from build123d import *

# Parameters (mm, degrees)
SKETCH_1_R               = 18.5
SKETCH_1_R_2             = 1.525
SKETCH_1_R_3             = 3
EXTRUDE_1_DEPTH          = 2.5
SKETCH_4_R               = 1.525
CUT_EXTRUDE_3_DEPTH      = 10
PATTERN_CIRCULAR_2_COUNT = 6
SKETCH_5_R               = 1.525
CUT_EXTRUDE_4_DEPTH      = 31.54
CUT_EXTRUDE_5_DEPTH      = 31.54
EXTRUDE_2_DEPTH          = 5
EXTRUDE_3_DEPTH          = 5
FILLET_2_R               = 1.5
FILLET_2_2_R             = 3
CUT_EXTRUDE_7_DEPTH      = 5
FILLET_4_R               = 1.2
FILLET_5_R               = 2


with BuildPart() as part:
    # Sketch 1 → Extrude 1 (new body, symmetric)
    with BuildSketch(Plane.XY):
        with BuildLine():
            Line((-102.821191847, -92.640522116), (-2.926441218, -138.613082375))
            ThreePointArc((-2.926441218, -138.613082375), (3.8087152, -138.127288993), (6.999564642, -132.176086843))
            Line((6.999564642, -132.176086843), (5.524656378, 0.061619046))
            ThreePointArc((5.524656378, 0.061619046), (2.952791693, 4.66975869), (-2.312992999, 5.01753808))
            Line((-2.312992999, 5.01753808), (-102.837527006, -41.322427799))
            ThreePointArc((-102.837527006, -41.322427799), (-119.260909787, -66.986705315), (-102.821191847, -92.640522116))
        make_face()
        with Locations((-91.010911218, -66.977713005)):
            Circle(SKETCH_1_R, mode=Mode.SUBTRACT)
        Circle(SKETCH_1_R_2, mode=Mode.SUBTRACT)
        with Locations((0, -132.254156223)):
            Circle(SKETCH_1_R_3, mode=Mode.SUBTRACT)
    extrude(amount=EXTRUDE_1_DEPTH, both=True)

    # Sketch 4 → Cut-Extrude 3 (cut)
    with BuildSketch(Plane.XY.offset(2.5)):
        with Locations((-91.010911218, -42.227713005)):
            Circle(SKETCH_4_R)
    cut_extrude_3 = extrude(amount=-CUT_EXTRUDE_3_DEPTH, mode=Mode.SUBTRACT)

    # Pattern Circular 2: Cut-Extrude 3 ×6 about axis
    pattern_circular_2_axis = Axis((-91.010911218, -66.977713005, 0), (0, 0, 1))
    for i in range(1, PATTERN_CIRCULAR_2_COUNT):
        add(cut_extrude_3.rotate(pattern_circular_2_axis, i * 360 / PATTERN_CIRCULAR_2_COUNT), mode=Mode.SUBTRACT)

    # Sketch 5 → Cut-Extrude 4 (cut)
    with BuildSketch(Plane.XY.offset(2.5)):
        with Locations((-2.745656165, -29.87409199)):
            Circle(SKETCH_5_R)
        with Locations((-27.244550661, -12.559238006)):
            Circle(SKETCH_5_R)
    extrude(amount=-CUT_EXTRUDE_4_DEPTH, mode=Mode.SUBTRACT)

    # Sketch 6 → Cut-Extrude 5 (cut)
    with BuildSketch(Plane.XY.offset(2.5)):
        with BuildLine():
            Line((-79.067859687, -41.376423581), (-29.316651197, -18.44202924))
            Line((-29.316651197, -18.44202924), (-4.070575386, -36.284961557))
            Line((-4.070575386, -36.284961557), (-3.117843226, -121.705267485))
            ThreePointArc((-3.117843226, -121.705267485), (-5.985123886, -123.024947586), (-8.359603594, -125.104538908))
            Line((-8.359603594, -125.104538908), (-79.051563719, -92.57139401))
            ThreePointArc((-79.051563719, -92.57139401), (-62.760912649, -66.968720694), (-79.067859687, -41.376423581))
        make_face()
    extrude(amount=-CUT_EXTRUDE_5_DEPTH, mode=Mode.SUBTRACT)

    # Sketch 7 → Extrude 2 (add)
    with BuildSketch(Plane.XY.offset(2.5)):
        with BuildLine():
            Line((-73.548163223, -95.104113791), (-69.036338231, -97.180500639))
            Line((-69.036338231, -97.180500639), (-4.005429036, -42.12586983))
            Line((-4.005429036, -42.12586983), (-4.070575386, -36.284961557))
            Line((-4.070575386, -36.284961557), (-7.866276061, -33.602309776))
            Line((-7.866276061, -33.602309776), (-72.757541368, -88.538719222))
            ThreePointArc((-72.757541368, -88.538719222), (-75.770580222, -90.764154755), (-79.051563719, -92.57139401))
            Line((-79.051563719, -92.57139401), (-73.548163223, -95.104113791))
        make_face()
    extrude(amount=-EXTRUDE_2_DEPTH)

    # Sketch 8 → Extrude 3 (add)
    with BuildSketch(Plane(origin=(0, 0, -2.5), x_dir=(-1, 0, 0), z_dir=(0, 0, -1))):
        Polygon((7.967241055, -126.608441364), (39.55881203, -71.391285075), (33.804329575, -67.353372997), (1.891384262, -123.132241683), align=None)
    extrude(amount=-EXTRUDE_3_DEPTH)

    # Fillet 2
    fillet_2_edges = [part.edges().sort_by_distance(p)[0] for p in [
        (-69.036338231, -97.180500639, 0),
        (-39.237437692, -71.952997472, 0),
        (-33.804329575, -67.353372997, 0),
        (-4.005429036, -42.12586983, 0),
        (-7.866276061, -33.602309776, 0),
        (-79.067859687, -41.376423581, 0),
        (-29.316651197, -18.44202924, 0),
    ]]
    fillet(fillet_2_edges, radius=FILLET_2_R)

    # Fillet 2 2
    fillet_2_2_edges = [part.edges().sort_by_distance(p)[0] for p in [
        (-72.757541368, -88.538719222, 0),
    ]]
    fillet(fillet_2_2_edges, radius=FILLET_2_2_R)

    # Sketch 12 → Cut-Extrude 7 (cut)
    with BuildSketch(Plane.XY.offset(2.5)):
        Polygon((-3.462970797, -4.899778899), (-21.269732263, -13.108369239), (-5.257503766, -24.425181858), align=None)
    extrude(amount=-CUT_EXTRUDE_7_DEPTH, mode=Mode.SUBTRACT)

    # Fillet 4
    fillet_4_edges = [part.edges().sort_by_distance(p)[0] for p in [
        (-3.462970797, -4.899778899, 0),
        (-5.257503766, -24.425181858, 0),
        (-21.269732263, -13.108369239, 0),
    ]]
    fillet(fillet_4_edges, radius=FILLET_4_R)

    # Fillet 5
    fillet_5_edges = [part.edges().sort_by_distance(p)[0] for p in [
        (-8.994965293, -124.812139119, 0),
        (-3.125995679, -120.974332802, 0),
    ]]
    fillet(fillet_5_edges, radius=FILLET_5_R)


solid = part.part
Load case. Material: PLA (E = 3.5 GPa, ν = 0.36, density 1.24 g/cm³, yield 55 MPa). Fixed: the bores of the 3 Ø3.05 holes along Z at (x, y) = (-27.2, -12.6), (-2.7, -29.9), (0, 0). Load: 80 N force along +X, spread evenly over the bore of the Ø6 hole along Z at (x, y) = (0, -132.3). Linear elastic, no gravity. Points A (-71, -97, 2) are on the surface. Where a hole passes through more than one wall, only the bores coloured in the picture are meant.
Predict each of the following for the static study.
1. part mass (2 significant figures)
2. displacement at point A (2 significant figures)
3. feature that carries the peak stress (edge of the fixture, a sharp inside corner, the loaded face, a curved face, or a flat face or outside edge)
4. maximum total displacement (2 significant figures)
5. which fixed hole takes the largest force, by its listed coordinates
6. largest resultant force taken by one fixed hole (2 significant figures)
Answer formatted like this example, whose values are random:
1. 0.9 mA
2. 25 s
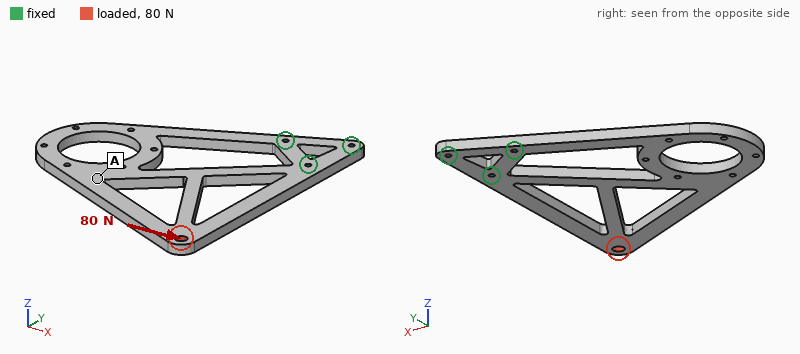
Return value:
1. 38 g
2. 1.8 mm
3. a curved face
4. 2.1 mm
5. (-2.7, -29.9)
6. 210 N
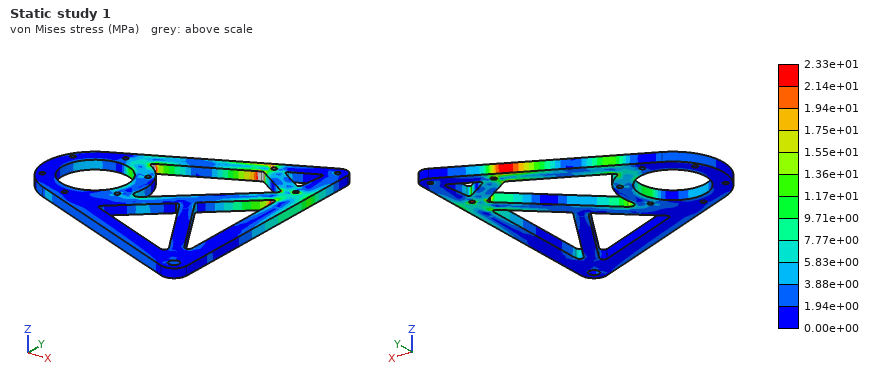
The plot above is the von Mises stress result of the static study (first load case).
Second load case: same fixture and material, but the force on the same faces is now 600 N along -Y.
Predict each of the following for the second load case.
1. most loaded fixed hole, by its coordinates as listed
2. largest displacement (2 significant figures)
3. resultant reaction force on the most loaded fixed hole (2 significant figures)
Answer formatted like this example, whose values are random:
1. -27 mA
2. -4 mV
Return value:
1. (-2.7, -29.9)
2. 0.42 mm
3. 530 N
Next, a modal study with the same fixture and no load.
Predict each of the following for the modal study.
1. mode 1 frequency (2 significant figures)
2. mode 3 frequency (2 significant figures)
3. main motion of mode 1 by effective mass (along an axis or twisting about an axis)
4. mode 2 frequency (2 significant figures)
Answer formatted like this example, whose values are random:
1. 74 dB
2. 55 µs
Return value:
1. 72 Hz
2. 240 Hz
3. along Z
4. 120 Hz
